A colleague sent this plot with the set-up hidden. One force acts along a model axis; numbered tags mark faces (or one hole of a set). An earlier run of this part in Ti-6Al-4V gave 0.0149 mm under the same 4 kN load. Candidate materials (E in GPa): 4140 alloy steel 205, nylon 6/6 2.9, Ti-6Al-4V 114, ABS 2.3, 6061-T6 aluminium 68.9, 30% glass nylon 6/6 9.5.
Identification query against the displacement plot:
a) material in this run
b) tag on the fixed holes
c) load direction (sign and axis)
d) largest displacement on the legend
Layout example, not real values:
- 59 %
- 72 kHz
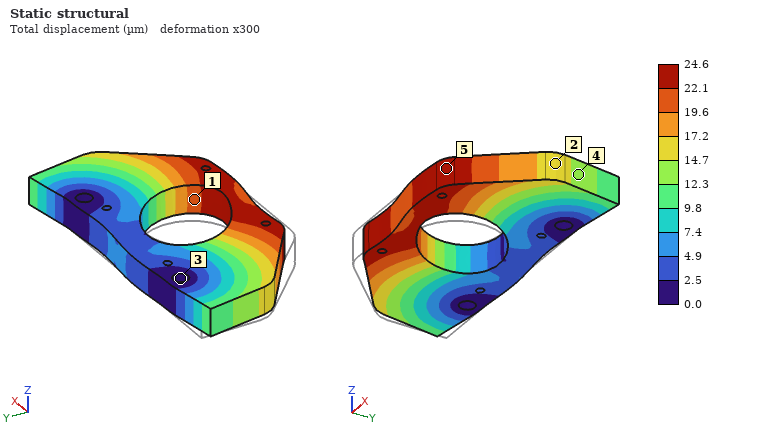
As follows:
- 6061-T6 aluminium
- 3
- +X
- 24.6 µm
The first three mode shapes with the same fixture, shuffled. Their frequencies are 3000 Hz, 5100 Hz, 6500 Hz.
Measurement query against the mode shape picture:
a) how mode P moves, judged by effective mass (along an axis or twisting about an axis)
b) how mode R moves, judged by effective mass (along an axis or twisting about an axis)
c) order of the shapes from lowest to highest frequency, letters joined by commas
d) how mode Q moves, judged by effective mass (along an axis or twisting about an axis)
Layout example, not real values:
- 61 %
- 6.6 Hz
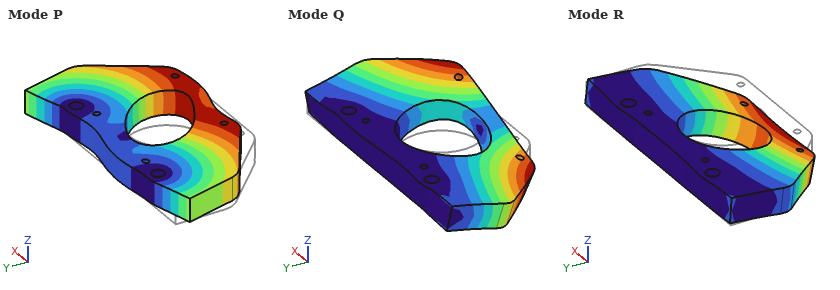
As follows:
- along X
- along Z
- R, Q, P
- twisting about Y
